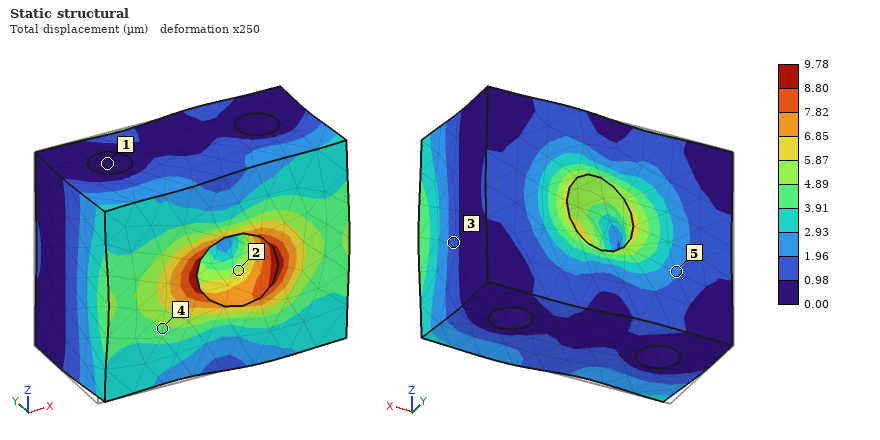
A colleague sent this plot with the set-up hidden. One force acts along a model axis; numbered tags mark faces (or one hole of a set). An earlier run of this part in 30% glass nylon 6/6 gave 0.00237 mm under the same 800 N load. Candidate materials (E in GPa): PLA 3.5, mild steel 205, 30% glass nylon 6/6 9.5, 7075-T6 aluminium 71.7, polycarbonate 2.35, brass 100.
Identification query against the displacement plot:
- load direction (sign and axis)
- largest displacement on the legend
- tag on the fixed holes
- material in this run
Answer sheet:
+X
9.78 µm
1
polycarbonate
